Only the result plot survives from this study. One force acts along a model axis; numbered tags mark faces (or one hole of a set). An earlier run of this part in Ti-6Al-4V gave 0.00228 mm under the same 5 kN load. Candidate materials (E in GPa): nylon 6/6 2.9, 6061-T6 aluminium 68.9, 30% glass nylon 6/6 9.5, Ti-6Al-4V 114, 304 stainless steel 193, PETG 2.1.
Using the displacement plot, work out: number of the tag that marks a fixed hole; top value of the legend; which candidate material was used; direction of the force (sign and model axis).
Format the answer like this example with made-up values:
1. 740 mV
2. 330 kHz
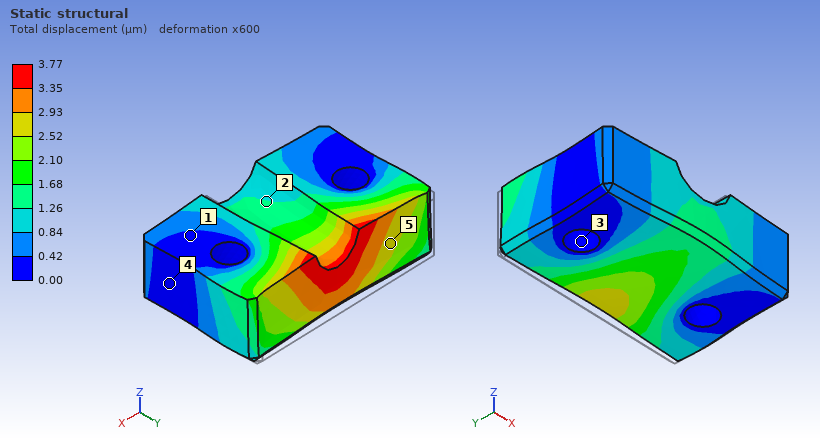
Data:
1. 3
2. 3.77 µm
3. 6061-T6 aluminium
4. -Y
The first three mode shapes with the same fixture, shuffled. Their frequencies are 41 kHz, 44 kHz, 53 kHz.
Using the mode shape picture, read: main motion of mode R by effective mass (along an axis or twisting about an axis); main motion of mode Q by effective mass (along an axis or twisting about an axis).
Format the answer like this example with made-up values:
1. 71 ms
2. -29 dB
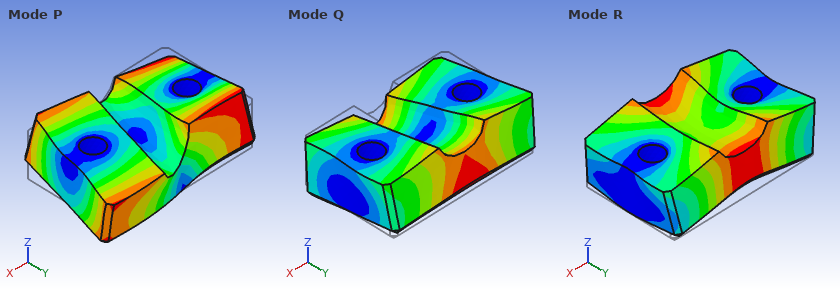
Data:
1. along Z
2. twisting about X
